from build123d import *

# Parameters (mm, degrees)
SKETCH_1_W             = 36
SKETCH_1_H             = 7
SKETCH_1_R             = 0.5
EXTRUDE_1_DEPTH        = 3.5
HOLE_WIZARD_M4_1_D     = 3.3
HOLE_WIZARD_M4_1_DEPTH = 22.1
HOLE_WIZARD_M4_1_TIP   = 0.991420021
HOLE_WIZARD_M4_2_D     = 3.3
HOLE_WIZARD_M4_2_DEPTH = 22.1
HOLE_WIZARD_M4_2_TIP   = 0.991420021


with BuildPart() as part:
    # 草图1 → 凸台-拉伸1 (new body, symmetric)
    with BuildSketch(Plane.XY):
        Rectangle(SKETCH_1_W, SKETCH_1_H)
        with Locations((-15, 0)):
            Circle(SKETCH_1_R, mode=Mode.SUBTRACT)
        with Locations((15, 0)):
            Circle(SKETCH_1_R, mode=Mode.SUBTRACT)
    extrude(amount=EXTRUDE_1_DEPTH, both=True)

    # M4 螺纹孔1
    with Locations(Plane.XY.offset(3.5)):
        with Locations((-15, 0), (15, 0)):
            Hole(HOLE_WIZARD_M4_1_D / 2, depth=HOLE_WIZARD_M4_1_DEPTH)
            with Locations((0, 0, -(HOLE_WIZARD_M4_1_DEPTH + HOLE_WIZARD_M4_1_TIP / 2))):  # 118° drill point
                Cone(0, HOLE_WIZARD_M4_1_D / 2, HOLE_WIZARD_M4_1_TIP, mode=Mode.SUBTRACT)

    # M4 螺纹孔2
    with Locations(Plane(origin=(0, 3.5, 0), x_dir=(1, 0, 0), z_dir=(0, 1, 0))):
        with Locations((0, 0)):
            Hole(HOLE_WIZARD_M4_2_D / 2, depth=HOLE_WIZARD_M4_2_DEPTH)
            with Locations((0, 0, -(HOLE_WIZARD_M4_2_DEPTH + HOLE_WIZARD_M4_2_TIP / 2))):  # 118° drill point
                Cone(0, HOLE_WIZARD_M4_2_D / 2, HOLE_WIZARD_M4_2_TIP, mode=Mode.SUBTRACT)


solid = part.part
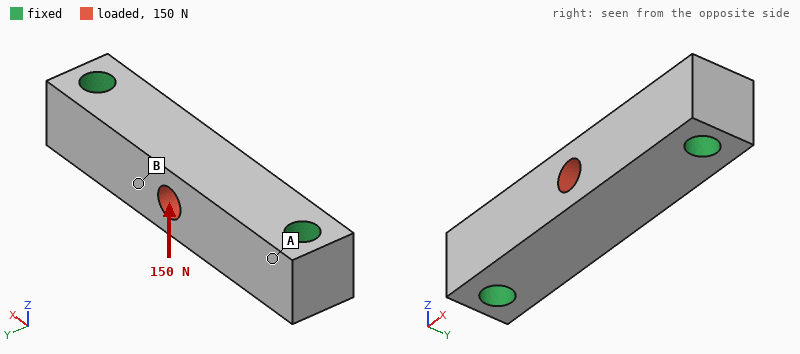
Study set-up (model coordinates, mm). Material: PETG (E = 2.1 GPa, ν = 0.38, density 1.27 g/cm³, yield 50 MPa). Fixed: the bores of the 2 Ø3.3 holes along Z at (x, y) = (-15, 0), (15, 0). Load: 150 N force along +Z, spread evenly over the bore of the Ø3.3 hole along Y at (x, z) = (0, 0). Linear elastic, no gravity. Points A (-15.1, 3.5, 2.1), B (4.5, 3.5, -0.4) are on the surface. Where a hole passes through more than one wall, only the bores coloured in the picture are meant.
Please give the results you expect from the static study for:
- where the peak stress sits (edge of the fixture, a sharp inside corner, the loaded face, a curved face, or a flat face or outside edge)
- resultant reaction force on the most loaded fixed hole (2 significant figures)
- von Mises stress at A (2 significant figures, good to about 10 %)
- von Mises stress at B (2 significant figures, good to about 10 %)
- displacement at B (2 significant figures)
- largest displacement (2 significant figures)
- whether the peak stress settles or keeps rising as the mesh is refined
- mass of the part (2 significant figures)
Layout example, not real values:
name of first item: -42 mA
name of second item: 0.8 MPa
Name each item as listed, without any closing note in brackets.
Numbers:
where the peak stress sits: edge of the fixture
resultant reaction force on the most loaded fixed hole: 75 N
von Mises stress at A: 2.0 MPa
von Mises stress at B: 4.5 MPa
displacement at B: 55 µm
largest displacement: 75 µm
whether the peak stress settles or keeps rising as the mesh is refined: keeps rising
mass of the part: 2.0 g
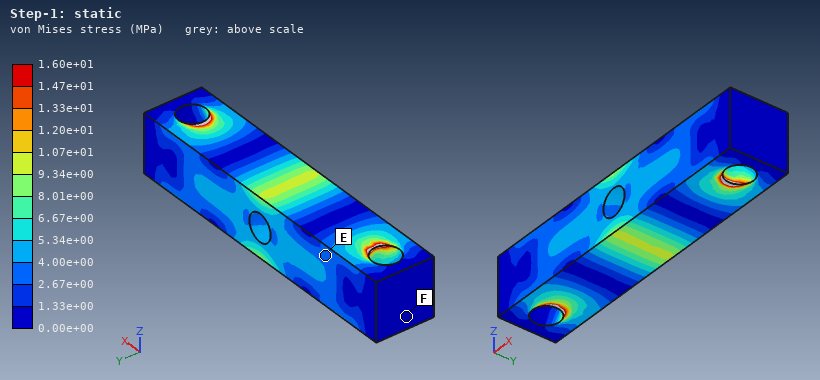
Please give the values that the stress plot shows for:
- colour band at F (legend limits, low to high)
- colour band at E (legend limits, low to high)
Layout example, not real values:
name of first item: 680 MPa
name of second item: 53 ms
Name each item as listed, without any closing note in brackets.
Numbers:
colour band at F: 0.00e+00 to 1.33e+00 MPa
colour band at E: 2.67e+00 to 4.00e+00 MPa
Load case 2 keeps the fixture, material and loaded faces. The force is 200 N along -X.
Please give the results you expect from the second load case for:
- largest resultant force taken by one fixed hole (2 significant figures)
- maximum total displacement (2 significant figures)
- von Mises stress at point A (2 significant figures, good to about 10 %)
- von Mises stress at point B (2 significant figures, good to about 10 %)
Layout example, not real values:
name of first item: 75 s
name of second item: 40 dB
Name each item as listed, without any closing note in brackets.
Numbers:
largest resultant force taken by one fixed hole: 100 N
maximum total displacement: 15 µm
von Mises stress at point A: 0.79 MPa
von Mises stress at point B: 2.5 MPa
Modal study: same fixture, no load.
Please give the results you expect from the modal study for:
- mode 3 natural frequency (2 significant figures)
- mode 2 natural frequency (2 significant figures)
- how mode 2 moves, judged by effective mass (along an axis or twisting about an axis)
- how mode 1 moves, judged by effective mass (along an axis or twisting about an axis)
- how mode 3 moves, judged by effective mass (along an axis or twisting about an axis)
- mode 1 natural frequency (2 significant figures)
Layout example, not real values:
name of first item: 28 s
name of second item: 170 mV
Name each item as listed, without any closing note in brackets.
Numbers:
mode 3 natural frequency: 13 kHz
mode 2 natural frequency: 9000 Hz
how mode 2 moves, judged by effective mass: along Z
how mode 1 moves, judged by effective mass: along Y
how mode 3 moves, judged by effective mass: twisting about X
mode 1 natural frequency: 7600 Hz
